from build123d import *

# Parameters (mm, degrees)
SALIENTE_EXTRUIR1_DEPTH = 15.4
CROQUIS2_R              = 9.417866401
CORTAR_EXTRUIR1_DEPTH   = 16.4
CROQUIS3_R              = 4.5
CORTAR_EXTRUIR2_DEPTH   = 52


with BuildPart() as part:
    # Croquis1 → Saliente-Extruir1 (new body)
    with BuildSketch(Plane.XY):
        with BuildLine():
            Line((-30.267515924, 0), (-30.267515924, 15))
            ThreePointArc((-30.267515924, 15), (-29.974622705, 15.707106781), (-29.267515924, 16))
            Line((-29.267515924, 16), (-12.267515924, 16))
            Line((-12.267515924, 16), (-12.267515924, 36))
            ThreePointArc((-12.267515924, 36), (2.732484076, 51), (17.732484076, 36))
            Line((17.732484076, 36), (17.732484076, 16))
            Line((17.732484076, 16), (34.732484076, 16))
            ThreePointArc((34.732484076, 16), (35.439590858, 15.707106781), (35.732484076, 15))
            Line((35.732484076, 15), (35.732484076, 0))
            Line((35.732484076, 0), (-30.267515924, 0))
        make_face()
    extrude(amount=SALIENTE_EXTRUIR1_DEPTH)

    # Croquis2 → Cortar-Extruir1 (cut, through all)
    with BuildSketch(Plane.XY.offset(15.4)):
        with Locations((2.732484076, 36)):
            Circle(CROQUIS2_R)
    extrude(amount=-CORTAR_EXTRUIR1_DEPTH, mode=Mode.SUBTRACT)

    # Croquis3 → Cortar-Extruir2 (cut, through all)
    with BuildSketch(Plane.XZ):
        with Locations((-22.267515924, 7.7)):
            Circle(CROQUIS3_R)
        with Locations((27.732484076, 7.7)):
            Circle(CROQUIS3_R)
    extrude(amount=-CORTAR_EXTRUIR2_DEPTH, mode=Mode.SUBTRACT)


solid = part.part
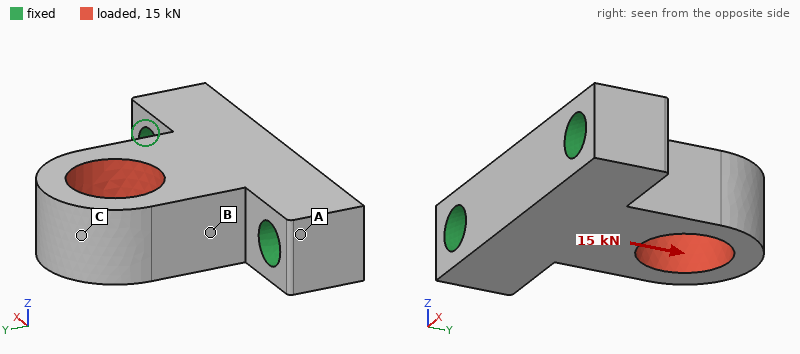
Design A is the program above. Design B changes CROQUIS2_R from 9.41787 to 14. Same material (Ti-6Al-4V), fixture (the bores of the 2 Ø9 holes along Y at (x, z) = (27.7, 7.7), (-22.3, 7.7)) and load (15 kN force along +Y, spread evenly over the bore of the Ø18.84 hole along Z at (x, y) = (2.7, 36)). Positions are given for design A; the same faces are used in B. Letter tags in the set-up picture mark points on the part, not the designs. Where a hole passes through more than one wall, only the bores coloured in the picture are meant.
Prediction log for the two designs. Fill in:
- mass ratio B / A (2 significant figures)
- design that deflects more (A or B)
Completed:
0.79
B
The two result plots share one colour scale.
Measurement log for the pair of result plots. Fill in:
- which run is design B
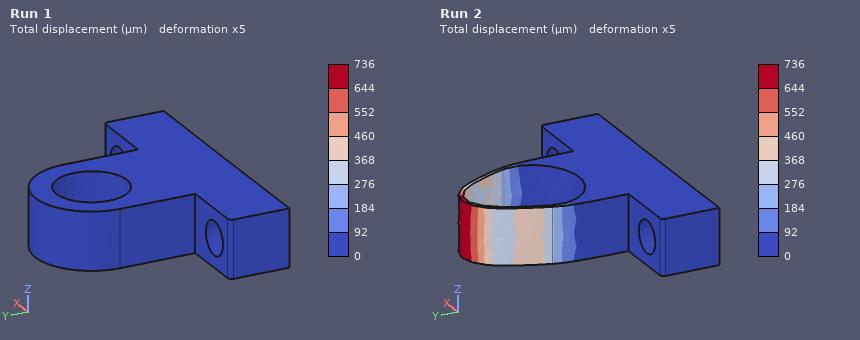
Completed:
Run 2
